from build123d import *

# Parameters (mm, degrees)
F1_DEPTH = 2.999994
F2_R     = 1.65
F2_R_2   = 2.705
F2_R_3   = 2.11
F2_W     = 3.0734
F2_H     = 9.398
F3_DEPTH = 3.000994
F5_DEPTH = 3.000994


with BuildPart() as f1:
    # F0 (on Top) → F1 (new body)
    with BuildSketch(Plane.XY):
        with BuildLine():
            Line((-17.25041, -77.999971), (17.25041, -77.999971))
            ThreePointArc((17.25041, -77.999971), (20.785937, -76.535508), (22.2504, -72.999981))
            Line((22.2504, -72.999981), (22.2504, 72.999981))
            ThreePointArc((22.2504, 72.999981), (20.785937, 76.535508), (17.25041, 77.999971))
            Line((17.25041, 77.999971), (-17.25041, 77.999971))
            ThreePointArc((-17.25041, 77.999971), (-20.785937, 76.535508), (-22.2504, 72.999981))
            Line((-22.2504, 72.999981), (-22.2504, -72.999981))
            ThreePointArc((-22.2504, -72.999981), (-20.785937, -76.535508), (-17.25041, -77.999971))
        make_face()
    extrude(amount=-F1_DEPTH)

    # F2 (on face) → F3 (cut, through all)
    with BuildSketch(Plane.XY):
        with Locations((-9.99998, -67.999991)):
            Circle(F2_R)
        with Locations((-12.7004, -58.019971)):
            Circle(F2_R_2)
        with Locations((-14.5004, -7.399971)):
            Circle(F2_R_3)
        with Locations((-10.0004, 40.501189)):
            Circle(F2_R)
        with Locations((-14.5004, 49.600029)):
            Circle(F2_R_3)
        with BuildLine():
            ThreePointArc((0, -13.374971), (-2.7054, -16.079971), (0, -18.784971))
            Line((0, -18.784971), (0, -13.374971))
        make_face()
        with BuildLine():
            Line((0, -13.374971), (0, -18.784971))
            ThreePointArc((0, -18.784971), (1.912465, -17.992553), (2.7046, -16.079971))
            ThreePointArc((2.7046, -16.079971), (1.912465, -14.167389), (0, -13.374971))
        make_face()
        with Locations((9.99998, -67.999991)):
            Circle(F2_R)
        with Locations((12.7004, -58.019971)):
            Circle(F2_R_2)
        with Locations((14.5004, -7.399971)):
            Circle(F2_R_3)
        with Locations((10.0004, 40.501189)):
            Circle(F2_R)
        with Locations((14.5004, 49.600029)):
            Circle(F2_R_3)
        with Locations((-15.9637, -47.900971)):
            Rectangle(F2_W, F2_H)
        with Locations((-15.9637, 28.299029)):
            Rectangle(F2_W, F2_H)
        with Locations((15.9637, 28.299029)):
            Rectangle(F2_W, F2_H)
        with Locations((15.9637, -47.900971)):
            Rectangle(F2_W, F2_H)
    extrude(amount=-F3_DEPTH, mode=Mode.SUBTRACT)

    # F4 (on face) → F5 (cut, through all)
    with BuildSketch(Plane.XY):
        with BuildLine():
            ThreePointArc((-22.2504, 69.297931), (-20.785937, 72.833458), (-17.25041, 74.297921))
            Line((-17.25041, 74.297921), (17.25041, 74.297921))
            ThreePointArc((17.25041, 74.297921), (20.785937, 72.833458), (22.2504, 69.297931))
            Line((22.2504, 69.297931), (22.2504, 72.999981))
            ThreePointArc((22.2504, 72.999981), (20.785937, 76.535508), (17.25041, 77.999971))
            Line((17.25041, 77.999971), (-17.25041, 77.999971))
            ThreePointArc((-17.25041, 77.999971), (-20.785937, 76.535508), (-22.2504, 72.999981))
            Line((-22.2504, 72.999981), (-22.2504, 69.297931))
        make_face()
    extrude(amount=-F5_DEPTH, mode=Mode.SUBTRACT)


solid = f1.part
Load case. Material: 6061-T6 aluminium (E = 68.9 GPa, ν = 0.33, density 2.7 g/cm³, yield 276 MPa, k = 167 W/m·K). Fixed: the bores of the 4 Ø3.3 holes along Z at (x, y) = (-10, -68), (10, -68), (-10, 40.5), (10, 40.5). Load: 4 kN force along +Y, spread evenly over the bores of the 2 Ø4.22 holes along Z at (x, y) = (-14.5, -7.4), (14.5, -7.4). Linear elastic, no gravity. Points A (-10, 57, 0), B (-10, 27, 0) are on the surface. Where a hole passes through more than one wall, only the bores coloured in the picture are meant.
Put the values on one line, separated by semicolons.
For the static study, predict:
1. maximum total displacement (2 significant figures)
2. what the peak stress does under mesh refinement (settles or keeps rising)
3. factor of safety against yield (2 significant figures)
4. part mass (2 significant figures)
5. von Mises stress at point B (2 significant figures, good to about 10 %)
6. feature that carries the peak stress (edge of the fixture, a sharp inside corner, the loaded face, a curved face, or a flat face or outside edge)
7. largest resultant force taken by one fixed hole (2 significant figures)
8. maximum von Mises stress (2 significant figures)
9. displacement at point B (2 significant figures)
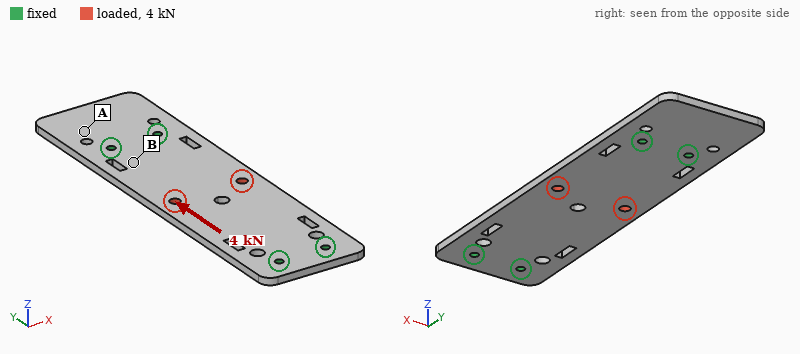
17 µm; settles; 3.1; 52 g; 20 MPa; the loaded face; 1.1 kN; 88 MPa; 5.1 µm
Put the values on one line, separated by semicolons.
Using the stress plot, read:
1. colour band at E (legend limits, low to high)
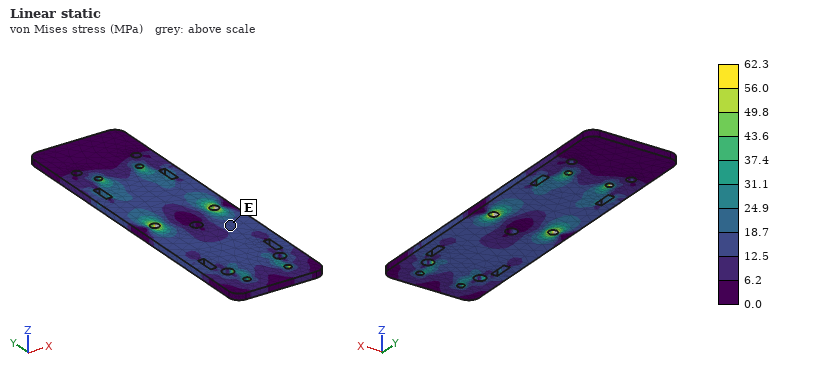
12.5 to 18.7 MPa
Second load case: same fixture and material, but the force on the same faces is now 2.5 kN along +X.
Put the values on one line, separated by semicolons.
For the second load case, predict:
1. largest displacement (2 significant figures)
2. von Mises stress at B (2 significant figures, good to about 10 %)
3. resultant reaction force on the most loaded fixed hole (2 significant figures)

45 µm; 28 MPa; 1.5 kN
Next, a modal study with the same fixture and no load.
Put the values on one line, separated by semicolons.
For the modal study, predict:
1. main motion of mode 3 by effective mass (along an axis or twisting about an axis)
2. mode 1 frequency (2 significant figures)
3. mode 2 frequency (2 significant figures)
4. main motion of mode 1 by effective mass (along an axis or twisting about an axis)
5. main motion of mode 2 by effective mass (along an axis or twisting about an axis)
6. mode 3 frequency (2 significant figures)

twisting about Y; 1300 Hz; 2100 Hz; along Z; along Z; 2300 Hz
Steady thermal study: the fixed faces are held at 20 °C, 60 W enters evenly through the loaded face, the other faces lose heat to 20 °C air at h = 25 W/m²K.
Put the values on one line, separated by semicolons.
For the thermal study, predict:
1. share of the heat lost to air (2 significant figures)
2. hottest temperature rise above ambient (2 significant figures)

16 %; 79 K
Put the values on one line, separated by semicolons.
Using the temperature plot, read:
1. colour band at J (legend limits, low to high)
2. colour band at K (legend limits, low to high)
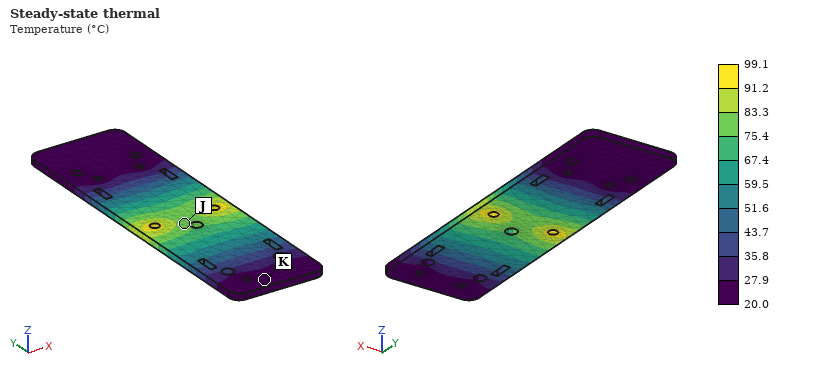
75.4 to 83.3 °C; 20.0 to 27.9 °C
